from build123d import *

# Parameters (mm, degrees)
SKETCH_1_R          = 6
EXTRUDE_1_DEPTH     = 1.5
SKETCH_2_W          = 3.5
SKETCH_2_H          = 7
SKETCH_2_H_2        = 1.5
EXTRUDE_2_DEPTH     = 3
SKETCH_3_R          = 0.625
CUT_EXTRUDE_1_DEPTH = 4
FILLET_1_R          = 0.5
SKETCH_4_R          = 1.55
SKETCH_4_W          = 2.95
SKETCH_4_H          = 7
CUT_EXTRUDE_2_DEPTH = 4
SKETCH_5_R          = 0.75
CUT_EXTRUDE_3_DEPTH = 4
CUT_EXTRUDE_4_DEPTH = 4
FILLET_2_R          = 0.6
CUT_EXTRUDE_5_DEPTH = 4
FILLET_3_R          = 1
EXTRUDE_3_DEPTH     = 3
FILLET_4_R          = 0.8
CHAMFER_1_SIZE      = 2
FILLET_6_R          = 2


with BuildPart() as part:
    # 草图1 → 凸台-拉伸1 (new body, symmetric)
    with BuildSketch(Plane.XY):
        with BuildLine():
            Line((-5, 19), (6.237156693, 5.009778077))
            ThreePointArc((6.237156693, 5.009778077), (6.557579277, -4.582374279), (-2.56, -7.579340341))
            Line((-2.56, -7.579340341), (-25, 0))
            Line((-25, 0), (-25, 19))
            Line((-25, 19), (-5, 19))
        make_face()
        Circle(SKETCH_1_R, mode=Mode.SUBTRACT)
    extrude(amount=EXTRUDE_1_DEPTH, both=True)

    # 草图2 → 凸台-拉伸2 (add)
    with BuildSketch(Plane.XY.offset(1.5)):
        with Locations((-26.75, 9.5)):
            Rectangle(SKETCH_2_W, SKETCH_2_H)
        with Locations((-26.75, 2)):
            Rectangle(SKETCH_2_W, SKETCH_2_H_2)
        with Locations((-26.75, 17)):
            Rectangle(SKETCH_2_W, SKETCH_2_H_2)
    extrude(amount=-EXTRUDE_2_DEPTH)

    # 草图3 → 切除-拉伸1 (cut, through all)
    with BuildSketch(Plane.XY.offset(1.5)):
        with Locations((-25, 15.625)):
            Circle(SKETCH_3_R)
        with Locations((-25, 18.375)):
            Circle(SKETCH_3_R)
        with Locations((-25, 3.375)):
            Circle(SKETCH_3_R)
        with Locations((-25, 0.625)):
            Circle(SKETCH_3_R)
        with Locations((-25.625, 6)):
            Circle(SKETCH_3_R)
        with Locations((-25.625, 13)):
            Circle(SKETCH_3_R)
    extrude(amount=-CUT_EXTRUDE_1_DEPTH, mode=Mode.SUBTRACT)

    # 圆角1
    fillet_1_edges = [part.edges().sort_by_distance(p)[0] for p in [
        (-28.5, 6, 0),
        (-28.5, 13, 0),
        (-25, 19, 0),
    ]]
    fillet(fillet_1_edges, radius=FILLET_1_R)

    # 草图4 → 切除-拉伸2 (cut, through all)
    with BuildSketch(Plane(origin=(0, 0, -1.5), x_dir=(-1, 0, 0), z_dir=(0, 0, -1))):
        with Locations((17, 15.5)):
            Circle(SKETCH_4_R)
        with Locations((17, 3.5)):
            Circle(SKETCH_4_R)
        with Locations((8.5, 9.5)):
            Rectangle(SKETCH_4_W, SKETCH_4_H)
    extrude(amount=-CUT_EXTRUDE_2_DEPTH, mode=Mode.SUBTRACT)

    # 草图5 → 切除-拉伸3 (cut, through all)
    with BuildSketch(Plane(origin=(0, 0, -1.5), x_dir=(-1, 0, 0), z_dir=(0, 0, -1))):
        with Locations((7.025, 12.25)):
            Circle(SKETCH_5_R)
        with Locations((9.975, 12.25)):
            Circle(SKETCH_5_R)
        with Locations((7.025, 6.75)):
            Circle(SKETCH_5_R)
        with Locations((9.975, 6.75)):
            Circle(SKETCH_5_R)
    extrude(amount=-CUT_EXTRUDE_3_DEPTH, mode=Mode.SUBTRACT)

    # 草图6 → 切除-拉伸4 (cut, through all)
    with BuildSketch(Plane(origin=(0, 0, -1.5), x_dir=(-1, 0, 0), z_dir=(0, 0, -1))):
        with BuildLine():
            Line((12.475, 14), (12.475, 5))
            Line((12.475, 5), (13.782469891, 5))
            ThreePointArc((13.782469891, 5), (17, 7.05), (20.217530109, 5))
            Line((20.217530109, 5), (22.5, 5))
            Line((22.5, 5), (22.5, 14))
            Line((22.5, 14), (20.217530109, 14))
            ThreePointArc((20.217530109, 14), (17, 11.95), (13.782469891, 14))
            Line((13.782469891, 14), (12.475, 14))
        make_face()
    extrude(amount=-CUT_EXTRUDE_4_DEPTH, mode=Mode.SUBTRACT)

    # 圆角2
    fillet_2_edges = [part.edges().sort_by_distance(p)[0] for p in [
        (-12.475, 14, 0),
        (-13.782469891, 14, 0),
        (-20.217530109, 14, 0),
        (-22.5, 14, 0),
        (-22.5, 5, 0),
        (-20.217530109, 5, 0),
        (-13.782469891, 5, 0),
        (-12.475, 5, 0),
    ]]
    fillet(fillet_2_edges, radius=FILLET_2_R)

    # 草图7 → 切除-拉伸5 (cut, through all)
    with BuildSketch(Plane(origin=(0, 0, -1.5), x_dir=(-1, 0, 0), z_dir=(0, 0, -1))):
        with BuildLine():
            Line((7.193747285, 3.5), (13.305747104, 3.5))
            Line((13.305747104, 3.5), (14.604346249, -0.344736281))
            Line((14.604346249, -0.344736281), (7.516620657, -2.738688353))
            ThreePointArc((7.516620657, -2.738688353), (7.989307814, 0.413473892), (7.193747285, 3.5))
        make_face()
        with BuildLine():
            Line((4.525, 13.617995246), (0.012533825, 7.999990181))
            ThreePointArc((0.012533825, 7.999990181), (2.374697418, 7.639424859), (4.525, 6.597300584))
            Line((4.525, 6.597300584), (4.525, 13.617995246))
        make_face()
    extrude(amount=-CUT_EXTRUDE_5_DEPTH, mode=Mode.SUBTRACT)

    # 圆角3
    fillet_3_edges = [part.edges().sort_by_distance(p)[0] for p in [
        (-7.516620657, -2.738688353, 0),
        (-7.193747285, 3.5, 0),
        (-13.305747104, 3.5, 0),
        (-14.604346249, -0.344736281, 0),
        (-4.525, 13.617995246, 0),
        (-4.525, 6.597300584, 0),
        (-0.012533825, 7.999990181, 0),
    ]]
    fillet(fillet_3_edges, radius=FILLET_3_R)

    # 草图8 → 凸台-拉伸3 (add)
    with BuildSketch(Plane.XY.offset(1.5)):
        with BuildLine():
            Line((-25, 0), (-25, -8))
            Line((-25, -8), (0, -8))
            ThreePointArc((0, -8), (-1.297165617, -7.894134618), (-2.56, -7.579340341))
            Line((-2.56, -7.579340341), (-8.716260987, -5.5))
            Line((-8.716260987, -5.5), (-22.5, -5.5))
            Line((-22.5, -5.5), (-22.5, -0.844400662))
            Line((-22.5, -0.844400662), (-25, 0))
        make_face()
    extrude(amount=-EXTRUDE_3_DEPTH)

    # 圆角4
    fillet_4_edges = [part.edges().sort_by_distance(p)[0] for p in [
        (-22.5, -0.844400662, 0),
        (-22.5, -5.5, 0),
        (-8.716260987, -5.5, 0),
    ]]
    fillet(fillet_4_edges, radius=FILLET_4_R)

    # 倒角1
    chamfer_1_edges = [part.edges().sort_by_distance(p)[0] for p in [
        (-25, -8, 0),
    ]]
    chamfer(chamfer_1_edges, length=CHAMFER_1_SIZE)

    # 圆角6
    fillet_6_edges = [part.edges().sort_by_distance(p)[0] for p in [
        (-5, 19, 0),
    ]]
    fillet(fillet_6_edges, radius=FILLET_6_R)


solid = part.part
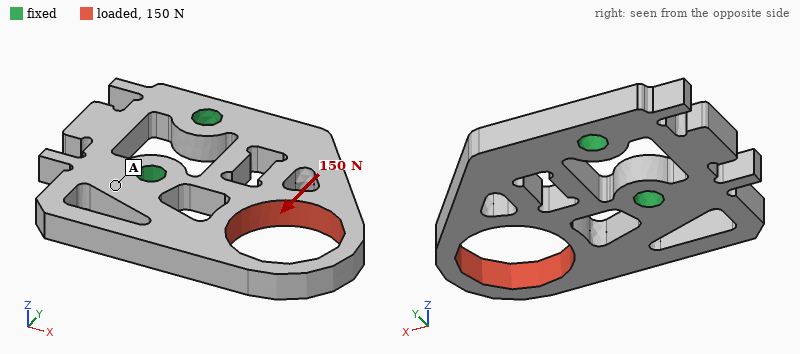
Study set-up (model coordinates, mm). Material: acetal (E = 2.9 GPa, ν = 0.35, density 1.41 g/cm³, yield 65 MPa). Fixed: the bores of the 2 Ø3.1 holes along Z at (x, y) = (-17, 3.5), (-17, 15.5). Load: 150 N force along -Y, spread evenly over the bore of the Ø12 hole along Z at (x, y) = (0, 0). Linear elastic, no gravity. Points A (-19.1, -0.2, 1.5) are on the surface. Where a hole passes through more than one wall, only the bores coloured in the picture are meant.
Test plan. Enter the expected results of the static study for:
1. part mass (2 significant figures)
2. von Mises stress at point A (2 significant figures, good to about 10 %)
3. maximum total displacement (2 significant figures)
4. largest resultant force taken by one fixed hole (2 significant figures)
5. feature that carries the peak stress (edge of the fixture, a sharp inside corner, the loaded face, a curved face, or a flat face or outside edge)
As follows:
2.1 g
7.7 MPa
0.49 mm
140 N
a curved face
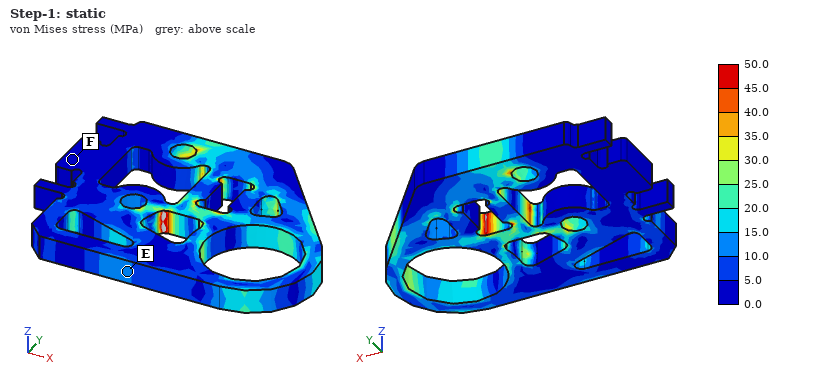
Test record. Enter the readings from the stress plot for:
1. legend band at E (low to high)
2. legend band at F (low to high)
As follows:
10.0 to 15.0 MPa
0.0 to 5.0 MPa
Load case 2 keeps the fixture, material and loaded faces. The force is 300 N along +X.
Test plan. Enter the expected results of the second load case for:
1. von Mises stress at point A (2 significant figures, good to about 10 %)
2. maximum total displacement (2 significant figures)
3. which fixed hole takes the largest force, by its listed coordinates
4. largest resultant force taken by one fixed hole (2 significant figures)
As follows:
12 MPa
0.43 mm
(-17, 3.5)
300 N
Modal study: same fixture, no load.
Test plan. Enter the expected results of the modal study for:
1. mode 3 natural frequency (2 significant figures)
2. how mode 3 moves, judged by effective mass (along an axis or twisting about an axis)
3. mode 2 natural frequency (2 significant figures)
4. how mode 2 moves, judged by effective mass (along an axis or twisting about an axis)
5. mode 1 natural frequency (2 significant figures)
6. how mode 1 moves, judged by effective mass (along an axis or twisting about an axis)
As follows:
3900 Hz
along Y
2600 Hz
twisting about X
1300 Hz
along Z
